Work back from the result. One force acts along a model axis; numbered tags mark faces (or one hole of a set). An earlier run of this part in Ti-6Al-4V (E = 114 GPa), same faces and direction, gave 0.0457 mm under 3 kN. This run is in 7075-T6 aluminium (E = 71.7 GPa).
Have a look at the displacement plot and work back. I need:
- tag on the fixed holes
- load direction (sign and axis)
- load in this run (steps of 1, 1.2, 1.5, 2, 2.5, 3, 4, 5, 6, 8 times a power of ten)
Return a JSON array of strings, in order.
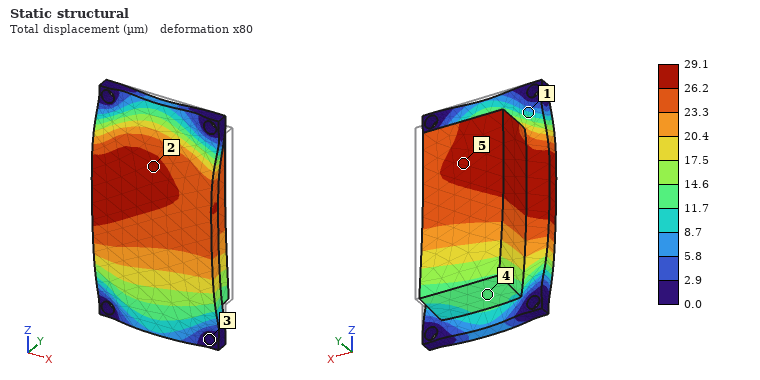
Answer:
["3", "-Y", "1.2 kN"]
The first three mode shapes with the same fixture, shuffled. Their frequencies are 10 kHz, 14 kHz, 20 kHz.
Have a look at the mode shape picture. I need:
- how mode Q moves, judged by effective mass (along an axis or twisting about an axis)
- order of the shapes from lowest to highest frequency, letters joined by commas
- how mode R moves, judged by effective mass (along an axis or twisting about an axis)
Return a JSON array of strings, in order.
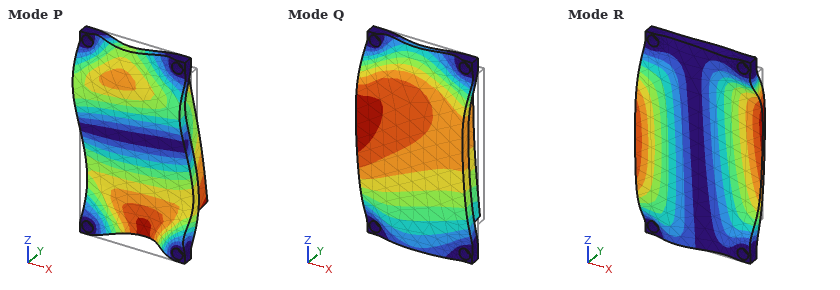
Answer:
["along Y", "Q, R, P", "along X"]
